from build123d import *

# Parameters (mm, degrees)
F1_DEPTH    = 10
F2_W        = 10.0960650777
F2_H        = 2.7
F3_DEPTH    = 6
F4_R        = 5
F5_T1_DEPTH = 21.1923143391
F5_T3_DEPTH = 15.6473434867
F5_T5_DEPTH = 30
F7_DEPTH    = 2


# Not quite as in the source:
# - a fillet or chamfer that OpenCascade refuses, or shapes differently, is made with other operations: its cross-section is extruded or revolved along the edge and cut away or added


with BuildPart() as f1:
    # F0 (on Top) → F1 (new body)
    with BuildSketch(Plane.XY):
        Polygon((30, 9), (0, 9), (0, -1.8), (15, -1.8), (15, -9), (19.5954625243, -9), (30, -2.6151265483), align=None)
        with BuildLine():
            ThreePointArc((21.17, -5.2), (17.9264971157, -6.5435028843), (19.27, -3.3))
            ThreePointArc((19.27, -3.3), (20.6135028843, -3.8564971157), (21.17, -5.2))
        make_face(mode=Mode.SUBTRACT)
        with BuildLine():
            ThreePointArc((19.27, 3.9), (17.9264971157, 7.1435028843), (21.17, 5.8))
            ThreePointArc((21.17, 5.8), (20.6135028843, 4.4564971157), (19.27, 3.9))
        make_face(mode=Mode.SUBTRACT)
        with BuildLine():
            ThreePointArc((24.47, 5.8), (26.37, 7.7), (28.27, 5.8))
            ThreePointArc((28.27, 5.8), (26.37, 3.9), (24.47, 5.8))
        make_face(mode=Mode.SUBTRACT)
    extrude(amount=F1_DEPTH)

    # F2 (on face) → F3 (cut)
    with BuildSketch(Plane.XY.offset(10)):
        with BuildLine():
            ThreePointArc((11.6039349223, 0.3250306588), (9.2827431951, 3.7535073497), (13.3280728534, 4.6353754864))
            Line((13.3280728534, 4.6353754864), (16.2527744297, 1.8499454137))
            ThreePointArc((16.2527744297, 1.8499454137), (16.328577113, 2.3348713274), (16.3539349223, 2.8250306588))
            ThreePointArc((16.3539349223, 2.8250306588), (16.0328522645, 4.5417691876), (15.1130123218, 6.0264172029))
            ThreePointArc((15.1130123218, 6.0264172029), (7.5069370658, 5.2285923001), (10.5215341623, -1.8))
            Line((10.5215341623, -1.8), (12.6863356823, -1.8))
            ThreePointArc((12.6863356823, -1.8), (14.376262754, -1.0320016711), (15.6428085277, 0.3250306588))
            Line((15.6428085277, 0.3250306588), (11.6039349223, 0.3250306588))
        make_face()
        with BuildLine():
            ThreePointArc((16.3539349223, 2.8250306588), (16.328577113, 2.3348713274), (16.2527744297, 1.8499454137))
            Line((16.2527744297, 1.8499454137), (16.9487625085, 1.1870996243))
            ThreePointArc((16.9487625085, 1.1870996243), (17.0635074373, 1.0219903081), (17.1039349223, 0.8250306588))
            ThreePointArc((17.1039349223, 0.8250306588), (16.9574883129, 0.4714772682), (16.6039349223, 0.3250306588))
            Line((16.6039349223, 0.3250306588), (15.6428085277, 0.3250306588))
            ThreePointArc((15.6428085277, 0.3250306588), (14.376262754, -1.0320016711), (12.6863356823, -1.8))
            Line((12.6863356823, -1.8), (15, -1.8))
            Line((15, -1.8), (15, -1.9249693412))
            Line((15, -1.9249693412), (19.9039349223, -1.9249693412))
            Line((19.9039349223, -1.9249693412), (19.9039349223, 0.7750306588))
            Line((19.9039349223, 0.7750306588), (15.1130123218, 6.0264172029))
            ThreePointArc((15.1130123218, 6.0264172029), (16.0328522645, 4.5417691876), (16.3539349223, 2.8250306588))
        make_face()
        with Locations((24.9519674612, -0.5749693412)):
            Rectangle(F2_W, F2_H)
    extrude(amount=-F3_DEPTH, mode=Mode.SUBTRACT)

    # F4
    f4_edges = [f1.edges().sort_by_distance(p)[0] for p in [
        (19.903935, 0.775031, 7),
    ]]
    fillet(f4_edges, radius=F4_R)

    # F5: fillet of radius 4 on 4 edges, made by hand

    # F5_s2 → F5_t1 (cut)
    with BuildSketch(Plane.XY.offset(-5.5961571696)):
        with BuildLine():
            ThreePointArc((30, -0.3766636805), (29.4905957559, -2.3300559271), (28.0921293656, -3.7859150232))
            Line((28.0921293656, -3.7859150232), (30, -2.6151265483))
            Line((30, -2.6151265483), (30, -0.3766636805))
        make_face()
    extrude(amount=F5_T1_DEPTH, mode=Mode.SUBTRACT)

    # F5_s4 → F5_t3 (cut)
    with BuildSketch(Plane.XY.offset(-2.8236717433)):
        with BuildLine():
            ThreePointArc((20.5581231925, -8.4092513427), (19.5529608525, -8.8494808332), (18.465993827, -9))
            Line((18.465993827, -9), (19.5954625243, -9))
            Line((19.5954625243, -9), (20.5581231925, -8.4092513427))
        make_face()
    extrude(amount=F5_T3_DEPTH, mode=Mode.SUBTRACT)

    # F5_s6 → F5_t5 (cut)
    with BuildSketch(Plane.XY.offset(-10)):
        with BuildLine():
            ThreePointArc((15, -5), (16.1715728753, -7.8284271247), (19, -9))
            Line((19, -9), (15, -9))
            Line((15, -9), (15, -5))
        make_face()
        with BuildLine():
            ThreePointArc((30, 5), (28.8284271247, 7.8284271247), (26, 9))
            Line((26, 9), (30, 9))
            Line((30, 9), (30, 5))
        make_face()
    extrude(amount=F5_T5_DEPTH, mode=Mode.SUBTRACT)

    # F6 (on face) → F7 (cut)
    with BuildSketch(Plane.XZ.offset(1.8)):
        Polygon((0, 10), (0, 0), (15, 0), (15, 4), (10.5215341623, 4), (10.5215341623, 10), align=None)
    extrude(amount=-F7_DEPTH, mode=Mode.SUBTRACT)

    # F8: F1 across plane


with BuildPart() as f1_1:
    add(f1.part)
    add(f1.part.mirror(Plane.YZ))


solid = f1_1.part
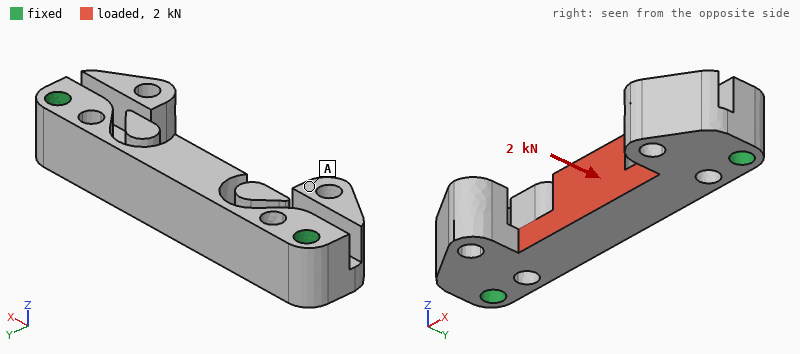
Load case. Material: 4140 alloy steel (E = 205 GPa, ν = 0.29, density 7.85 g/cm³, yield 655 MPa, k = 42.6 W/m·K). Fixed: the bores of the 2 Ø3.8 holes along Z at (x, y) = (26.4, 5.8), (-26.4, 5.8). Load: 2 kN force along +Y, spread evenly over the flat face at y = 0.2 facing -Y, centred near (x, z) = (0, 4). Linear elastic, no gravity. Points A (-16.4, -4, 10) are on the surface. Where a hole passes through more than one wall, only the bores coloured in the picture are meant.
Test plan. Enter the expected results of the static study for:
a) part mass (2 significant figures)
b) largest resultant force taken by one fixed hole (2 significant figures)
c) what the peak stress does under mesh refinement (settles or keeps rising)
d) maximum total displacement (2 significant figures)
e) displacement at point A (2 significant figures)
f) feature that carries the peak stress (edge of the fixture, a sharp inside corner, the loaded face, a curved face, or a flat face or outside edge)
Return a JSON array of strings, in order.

["44 g", "1.0 kN", "keeps rising", "28 µm", "10 µm", "a sharp inside corner"]
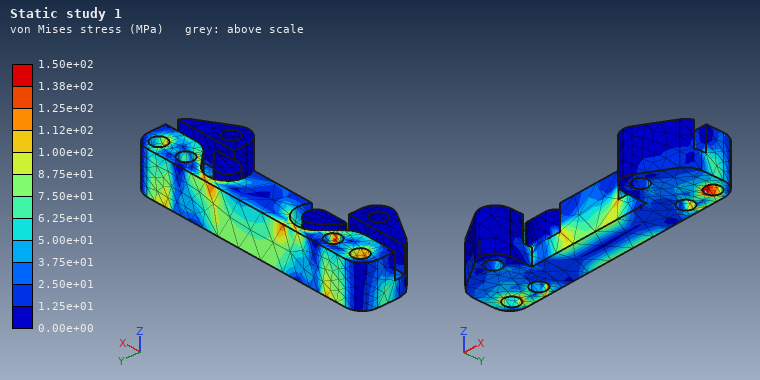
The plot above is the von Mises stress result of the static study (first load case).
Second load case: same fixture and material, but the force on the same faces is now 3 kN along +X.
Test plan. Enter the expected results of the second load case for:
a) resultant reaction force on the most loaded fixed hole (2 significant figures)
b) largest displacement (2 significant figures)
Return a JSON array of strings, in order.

["1.5 kN", "10 µm"]
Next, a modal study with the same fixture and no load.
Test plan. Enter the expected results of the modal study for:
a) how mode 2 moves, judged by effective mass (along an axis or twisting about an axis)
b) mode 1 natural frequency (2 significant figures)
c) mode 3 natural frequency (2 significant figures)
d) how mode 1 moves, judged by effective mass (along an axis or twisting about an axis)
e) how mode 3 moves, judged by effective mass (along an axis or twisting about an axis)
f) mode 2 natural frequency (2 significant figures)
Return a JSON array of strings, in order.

["along Z", "11 kHz", "15 kHz", "along Y", "twisting about X", "12 kHz"]
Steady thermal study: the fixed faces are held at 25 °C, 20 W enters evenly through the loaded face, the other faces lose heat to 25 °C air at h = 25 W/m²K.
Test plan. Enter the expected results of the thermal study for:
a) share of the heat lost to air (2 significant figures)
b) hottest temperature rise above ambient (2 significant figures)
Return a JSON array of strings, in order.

["13 %", "83 K"]
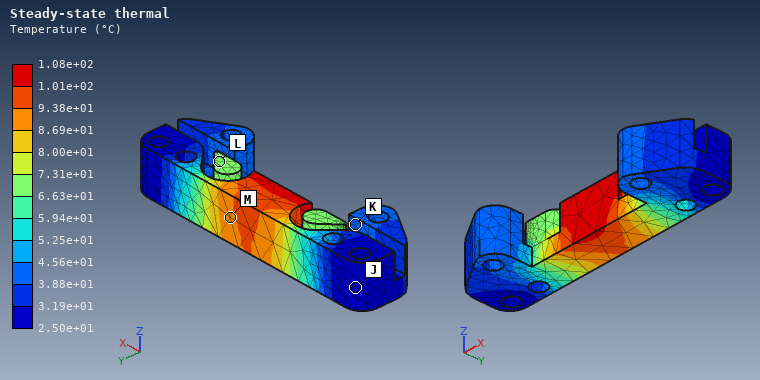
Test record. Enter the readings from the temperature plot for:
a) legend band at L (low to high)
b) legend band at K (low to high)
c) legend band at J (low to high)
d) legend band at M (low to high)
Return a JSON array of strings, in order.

["6.63e+01 to 7.31e+01 °C", "3.88e+01 to 4.56e+01 °C", "2.50e+01 to 3.19e+01 °C", "8.69e+01 to 9.38e+01 °C"]
